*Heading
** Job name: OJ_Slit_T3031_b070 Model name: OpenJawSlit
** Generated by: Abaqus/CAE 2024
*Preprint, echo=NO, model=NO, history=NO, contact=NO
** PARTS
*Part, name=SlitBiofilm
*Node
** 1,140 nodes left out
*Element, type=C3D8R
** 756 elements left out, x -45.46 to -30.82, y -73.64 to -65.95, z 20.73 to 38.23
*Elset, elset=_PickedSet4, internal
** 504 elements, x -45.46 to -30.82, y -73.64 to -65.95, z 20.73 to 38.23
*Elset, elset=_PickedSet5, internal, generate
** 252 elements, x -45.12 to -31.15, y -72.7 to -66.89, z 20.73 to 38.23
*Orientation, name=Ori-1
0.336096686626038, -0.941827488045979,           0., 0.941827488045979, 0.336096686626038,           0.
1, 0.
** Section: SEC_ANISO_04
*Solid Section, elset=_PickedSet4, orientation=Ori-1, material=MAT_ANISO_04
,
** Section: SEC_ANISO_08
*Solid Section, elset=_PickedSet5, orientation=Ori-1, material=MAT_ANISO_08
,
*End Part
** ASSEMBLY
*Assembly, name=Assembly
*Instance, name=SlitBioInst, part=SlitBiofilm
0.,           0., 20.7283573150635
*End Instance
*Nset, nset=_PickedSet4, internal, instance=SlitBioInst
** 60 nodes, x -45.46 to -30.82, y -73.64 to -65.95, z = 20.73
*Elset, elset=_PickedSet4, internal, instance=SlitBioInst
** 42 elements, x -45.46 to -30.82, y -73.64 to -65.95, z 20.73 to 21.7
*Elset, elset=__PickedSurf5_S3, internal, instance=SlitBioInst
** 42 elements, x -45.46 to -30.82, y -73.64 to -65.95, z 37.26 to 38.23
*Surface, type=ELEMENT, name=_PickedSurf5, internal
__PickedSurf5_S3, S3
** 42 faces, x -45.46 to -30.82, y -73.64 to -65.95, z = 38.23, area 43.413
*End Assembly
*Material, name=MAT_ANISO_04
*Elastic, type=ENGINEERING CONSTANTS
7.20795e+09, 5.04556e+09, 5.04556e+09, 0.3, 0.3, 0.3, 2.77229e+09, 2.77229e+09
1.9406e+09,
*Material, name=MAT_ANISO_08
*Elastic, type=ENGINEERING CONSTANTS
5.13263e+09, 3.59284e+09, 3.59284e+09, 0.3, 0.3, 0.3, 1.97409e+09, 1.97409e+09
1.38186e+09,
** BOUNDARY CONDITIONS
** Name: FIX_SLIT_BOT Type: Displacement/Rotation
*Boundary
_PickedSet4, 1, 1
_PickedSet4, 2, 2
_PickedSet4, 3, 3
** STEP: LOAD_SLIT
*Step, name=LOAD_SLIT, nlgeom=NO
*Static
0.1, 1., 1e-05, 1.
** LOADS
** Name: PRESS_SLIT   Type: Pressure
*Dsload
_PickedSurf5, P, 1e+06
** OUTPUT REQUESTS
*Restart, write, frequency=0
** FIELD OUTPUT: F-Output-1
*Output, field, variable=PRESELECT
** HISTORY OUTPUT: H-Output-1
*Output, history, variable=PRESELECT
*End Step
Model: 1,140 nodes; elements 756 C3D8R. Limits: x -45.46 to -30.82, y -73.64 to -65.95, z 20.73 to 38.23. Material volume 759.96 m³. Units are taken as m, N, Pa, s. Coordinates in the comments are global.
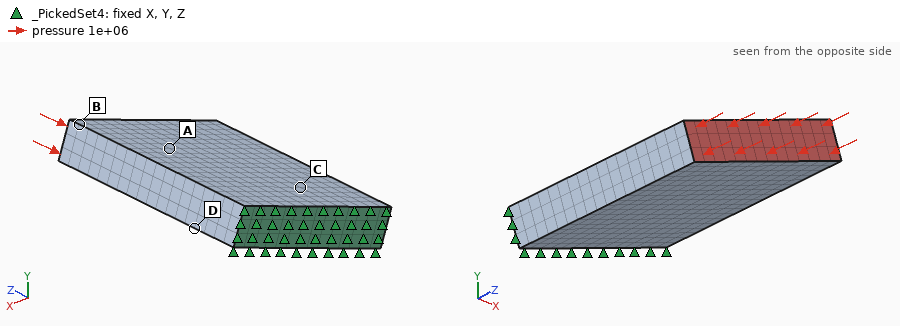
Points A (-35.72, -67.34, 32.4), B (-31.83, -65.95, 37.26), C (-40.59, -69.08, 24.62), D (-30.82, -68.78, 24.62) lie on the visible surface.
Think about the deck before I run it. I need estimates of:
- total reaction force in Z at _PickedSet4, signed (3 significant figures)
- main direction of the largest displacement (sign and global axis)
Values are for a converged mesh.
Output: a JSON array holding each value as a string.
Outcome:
["4.34e+07 N", "-Z"]
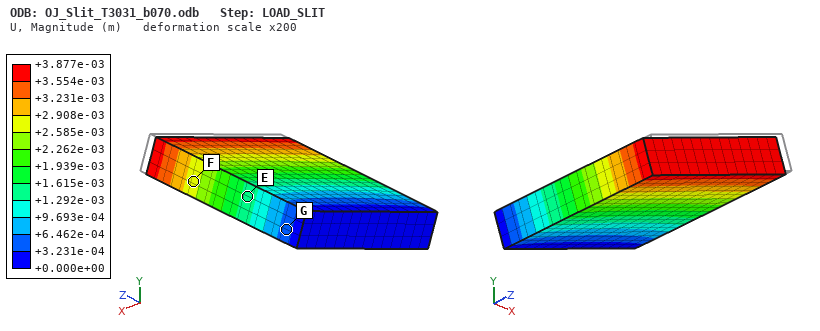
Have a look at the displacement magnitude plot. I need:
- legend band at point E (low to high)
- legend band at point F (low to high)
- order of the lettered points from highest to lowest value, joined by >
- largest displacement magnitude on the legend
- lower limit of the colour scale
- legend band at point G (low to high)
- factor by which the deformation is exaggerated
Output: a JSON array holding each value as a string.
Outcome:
["+1.292e-03 to +1.615e-03 m", "+2.585e-03 to +2.908e-03 m", "F > E > G", "+3.877e-03 m", "+0.000e+00 m", "+3.231e-04 to +6.462e-04 m", "200"]
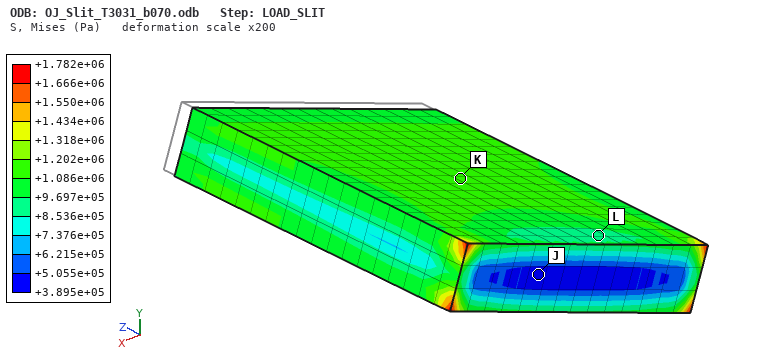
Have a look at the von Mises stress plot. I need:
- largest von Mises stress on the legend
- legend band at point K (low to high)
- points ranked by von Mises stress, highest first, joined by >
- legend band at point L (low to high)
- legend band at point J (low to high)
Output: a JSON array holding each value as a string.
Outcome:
["+1.782e+06 Pa", "+1.086e+06 to +1.202e+06 Pa", "K > L > J", "+8.536e+05 to +9.697e+05 Pa", "+3.895e+05 to +5.055e+05 Pa"]
